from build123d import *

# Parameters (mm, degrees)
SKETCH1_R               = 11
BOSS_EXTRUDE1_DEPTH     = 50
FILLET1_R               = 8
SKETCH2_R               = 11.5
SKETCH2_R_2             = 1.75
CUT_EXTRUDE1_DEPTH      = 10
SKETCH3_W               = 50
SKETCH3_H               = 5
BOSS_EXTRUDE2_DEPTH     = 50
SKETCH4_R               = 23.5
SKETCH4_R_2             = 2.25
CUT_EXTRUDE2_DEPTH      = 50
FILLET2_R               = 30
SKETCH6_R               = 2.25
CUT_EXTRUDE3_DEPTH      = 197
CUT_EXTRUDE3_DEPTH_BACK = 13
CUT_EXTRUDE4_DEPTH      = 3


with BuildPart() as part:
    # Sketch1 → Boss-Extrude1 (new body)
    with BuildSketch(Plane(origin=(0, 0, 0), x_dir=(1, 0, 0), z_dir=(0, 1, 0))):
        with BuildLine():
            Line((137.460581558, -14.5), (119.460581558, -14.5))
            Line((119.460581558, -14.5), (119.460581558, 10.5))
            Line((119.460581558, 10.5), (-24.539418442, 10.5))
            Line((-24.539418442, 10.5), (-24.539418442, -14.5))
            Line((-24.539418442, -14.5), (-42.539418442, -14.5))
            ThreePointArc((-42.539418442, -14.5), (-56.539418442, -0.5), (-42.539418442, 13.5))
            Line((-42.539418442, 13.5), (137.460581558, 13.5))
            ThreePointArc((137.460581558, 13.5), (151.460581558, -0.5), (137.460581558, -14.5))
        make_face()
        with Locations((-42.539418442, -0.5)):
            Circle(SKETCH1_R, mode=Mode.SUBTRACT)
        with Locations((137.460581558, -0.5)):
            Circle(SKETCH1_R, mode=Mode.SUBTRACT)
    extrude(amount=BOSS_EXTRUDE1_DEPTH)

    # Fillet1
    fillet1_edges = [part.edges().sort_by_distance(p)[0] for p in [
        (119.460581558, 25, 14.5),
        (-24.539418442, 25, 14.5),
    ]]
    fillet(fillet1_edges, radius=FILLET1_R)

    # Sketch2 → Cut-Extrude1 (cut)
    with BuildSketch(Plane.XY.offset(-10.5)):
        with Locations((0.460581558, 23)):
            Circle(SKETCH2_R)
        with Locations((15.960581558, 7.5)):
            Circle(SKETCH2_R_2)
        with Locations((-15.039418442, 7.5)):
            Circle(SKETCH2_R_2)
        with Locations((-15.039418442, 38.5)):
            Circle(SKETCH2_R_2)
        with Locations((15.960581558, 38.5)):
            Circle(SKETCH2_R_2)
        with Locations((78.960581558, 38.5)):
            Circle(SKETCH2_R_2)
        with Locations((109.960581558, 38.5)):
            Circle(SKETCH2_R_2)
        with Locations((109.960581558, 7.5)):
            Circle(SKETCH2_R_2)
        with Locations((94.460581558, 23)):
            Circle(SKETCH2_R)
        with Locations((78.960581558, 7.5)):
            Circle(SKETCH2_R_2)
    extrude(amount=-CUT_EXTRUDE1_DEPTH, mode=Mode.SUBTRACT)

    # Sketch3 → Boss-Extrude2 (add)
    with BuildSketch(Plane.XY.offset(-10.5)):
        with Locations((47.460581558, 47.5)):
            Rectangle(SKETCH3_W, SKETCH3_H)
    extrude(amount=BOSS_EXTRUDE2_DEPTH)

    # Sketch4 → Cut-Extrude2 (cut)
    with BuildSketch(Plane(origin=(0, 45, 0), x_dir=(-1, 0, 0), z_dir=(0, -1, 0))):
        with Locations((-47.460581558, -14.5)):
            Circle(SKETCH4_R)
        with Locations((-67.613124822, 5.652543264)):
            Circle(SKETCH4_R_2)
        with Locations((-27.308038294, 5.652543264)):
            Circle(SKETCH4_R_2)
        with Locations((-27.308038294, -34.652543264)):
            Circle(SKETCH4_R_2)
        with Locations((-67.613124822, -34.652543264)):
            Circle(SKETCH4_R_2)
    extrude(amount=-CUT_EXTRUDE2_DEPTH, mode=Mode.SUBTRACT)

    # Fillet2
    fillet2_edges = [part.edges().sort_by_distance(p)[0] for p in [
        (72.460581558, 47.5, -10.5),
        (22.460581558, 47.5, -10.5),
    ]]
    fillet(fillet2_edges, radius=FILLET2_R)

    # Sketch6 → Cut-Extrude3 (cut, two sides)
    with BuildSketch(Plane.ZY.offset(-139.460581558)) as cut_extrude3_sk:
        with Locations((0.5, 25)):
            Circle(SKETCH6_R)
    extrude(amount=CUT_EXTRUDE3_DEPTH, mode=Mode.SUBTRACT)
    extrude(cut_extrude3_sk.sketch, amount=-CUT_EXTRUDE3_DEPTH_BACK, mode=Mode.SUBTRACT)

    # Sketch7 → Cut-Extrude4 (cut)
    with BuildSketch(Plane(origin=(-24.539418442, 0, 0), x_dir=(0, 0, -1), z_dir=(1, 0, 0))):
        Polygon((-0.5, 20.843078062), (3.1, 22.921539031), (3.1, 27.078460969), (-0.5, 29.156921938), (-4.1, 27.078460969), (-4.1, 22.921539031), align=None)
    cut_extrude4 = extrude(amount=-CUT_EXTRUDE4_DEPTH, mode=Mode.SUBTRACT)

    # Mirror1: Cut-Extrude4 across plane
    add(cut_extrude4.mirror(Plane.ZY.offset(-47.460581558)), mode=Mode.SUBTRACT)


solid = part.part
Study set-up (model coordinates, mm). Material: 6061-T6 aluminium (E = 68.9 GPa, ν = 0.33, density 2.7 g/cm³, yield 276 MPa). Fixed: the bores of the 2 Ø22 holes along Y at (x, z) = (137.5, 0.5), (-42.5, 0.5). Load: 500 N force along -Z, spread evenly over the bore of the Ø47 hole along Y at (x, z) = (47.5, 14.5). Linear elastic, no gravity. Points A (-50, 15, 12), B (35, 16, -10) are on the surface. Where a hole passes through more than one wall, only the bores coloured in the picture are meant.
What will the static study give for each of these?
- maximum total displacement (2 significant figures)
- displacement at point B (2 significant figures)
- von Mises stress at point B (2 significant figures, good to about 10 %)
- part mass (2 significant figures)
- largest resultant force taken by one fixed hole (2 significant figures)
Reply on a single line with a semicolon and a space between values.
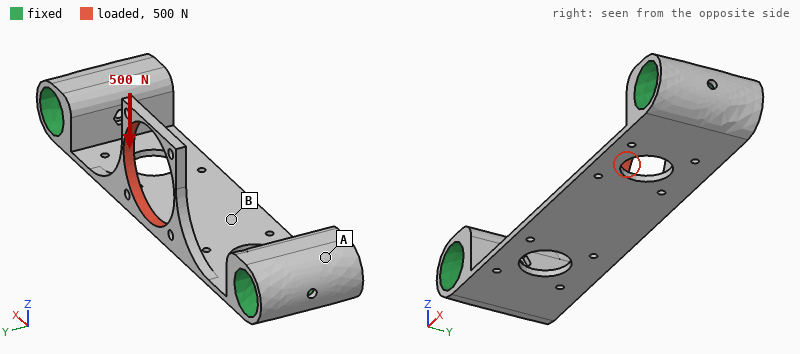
0.78 mm; 0.29 mm; 27 MPa; 180 g; 410 N
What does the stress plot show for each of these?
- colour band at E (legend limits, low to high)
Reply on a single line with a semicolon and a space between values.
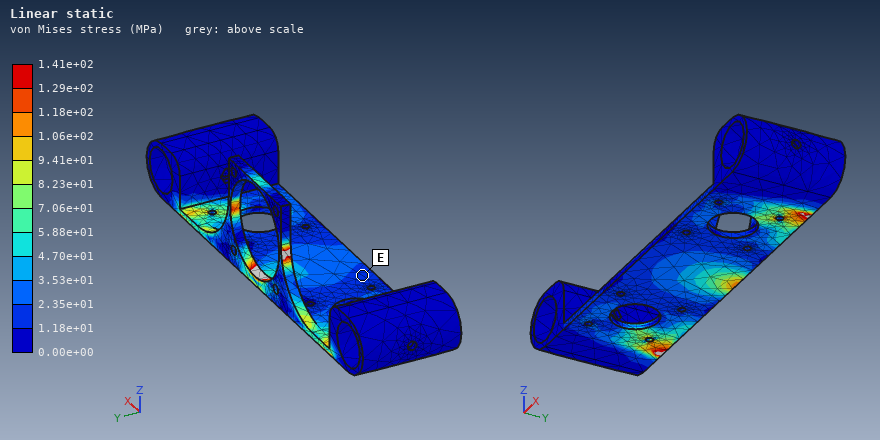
1.18e+01 to 2.35e+01 MPa
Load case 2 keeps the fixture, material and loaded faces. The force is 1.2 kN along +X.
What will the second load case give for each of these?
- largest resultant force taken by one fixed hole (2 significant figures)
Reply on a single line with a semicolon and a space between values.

670 N
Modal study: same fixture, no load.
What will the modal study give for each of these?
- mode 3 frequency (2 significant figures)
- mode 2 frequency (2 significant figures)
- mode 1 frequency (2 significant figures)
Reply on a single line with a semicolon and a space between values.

1700 Hz; 780 Hz; 770 Hz
